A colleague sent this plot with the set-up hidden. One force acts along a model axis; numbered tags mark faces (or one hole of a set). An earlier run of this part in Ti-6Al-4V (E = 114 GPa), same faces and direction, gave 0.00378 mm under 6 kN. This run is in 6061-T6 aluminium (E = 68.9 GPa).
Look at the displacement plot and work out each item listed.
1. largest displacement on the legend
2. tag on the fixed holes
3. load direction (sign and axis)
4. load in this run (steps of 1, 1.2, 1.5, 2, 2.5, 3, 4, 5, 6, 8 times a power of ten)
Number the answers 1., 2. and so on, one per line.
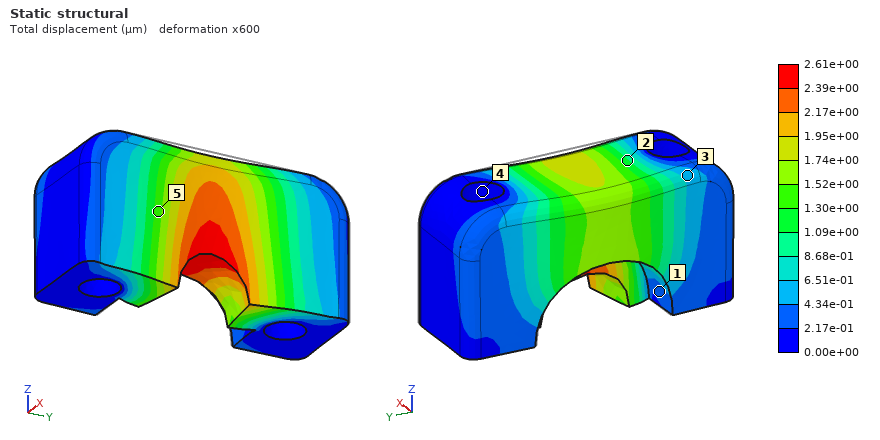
1. 2.61e+00 µm
2. 4
3. -X
4. 2.5 kN
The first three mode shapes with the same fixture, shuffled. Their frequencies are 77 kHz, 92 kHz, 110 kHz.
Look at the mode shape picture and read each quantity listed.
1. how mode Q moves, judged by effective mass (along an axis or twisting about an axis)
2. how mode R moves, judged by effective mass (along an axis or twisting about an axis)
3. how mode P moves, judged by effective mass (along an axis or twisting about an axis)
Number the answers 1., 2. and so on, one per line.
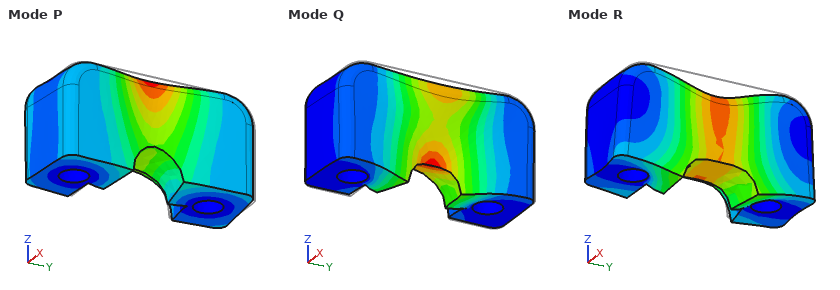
1. twisting about Y
2. along Z
3. along X
